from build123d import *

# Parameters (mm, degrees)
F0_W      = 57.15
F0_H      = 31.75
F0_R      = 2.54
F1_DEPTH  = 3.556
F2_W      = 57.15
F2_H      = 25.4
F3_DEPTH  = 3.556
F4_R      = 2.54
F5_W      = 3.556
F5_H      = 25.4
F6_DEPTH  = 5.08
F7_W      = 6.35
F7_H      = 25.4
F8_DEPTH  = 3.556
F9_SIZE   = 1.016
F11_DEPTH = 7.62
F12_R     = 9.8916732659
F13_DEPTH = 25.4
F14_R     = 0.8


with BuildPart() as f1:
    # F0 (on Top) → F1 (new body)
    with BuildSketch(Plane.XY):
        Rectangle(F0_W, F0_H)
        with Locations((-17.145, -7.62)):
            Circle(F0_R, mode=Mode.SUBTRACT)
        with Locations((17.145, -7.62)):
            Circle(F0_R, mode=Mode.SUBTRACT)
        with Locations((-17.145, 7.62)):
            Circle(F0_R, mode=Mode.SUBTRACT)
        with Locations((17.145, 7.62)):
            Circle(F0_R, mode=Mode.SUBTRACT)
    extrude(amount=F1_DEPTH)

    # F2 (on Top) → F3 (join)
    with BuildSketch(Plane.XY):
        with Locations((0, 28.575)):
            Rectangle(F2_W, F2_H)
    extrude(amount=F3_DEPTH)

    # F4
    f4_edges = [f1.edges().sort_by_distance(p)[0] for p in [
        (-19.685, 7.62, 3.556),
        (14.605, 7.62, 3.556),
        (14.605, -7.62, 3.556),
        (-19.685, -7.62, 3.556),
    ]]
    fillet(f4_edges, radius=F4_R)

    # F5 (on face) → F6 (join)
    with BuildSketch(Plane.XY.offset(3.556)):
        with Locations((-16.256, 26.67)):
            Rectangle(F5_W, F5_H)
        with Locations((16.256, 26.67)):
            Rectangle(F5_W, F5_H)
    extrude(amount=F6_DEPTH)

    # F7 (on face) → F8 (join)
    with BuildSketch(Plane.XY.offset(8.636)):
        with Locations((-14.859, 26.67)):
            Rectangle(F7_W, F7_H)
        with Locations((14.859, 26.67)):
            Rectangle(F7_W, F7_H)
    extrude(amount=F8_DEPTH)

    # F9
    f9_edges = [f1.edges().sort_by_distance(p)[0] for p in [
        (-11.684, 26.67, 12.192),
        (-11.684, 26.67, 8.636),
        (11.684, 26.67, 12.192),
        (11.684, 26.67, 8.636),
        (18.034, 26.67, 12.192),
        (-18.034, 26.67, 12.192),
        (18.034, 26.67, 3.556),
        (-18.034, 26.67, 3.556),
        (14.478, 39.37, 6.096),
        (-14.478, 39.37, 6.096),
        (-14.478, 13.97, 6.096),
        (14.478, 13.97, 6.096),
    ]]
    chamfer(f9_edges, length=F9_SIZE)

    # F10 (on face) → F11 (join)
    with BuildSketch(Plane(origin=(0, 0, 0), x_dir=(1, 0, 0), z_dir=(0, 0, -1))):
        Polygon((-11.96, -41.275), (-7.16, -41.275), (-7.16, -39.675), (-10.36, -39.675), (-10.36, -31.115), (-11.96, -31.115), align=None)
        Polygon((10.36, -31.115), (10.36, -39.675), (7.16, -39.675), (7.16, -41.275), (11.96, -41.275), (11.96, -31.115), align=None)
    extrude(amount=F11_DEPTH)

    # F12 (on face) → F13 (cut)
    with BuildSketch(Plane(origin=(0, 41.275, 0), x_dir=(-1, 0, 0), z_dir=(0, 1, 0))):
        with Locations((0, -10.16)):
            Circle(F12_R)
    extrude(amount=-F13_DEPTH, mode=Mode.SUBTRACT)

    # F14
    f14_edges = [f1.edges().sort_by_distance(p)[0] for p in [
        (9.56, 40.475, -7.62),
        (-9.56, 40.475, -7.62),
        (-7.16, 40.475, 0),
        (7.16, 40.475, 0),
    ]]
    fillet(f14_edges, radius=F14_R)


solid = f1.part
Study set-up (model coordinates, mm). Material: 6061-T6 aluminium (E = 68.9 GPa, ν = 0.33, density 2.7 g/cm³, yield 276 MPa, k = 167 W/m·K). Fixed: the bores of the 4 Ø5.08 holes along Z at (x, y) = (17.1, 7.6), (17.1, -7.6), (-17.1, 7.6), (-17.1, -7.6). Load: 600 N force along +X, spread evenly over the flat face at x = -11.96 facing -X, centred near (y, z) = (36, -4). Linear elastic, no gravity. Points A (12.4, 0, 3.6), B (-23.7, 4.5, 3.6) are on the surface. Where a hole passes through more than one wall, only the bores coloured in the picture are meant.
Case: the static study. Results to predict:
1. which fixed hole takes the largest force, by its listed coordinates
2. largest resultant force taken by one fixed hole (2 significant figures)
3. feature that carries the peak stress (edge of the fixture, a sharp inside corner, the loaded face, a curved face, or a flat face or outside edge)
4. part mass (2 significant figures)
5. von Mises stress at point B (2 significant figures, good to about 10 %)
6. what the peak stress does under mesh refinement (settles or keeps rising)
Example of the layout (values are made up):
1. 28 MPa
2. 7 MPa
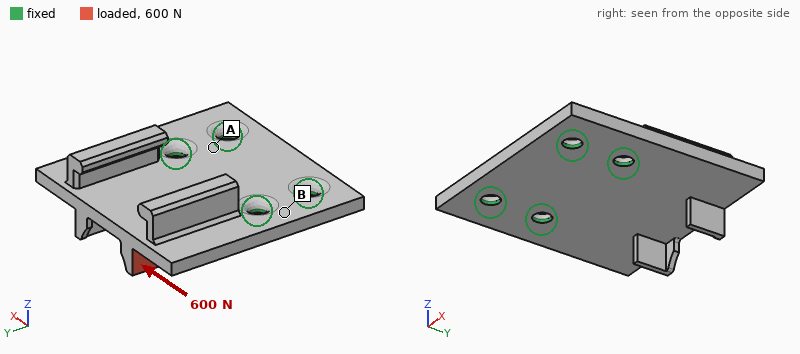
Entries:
1. (-17.1, 7.6)
2. 510 N
3. a sharp inside corner
4. 37 g
5. 29 MPa
6. keeps rising
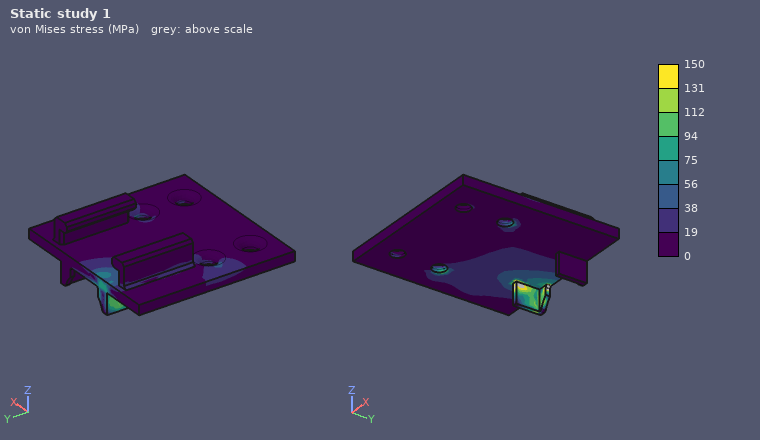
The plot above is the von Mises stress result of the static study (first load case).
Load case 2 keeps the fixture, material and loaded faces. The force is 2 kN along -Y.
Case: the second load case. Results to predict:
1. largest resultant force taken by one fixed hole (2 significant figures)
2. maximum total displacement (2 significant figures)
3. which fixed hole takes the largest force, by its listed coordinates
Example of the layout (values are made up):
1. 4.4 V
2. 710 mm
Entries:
1. 1.7 kN
2. 0.49 mm
3. (-17.1, 7.6)
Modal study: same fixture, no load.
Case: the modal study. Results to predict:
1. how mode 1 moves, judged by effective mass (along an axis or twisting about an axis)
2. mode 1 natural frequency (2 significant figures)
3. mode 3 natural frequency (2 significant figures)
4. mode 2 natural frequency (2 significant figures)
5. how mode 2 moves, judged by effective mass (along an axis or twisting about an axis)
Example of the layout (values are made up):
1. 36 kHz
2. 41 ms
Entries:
1. along Z
2. 1900 Hz
3. 6900 Hz
4. 3400 Hz
5. twisting about Y
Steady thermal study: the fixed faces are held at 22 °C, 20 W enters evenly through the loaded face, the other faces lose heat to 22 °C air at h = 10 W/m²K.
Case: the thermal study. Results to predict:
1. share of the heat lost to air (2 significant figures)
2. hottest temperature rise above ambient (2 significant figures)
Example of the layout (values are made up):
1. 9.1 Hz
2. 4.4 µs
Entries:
1. 3.7 %
2. 56 K
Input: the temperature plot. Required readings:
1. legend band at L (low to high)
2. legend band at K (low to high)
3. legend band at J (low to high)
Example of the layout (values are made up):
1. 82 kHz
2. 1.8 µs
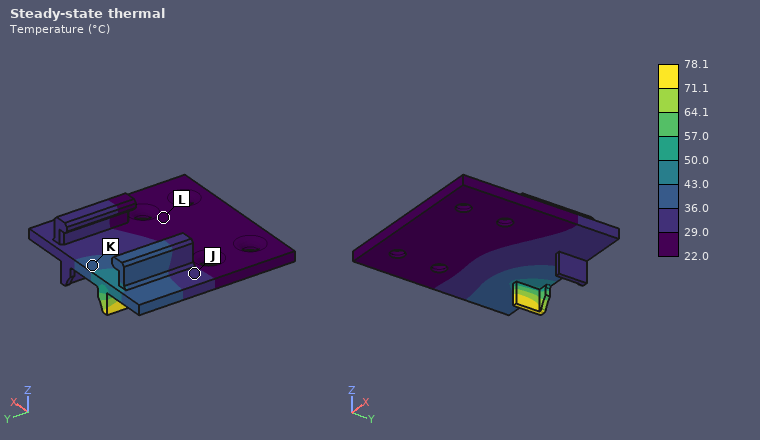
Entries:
1. 22.0 to 29.0 °C
2. 36.0 to 43.0 °C
3. 29.0 to 36.0 °C
